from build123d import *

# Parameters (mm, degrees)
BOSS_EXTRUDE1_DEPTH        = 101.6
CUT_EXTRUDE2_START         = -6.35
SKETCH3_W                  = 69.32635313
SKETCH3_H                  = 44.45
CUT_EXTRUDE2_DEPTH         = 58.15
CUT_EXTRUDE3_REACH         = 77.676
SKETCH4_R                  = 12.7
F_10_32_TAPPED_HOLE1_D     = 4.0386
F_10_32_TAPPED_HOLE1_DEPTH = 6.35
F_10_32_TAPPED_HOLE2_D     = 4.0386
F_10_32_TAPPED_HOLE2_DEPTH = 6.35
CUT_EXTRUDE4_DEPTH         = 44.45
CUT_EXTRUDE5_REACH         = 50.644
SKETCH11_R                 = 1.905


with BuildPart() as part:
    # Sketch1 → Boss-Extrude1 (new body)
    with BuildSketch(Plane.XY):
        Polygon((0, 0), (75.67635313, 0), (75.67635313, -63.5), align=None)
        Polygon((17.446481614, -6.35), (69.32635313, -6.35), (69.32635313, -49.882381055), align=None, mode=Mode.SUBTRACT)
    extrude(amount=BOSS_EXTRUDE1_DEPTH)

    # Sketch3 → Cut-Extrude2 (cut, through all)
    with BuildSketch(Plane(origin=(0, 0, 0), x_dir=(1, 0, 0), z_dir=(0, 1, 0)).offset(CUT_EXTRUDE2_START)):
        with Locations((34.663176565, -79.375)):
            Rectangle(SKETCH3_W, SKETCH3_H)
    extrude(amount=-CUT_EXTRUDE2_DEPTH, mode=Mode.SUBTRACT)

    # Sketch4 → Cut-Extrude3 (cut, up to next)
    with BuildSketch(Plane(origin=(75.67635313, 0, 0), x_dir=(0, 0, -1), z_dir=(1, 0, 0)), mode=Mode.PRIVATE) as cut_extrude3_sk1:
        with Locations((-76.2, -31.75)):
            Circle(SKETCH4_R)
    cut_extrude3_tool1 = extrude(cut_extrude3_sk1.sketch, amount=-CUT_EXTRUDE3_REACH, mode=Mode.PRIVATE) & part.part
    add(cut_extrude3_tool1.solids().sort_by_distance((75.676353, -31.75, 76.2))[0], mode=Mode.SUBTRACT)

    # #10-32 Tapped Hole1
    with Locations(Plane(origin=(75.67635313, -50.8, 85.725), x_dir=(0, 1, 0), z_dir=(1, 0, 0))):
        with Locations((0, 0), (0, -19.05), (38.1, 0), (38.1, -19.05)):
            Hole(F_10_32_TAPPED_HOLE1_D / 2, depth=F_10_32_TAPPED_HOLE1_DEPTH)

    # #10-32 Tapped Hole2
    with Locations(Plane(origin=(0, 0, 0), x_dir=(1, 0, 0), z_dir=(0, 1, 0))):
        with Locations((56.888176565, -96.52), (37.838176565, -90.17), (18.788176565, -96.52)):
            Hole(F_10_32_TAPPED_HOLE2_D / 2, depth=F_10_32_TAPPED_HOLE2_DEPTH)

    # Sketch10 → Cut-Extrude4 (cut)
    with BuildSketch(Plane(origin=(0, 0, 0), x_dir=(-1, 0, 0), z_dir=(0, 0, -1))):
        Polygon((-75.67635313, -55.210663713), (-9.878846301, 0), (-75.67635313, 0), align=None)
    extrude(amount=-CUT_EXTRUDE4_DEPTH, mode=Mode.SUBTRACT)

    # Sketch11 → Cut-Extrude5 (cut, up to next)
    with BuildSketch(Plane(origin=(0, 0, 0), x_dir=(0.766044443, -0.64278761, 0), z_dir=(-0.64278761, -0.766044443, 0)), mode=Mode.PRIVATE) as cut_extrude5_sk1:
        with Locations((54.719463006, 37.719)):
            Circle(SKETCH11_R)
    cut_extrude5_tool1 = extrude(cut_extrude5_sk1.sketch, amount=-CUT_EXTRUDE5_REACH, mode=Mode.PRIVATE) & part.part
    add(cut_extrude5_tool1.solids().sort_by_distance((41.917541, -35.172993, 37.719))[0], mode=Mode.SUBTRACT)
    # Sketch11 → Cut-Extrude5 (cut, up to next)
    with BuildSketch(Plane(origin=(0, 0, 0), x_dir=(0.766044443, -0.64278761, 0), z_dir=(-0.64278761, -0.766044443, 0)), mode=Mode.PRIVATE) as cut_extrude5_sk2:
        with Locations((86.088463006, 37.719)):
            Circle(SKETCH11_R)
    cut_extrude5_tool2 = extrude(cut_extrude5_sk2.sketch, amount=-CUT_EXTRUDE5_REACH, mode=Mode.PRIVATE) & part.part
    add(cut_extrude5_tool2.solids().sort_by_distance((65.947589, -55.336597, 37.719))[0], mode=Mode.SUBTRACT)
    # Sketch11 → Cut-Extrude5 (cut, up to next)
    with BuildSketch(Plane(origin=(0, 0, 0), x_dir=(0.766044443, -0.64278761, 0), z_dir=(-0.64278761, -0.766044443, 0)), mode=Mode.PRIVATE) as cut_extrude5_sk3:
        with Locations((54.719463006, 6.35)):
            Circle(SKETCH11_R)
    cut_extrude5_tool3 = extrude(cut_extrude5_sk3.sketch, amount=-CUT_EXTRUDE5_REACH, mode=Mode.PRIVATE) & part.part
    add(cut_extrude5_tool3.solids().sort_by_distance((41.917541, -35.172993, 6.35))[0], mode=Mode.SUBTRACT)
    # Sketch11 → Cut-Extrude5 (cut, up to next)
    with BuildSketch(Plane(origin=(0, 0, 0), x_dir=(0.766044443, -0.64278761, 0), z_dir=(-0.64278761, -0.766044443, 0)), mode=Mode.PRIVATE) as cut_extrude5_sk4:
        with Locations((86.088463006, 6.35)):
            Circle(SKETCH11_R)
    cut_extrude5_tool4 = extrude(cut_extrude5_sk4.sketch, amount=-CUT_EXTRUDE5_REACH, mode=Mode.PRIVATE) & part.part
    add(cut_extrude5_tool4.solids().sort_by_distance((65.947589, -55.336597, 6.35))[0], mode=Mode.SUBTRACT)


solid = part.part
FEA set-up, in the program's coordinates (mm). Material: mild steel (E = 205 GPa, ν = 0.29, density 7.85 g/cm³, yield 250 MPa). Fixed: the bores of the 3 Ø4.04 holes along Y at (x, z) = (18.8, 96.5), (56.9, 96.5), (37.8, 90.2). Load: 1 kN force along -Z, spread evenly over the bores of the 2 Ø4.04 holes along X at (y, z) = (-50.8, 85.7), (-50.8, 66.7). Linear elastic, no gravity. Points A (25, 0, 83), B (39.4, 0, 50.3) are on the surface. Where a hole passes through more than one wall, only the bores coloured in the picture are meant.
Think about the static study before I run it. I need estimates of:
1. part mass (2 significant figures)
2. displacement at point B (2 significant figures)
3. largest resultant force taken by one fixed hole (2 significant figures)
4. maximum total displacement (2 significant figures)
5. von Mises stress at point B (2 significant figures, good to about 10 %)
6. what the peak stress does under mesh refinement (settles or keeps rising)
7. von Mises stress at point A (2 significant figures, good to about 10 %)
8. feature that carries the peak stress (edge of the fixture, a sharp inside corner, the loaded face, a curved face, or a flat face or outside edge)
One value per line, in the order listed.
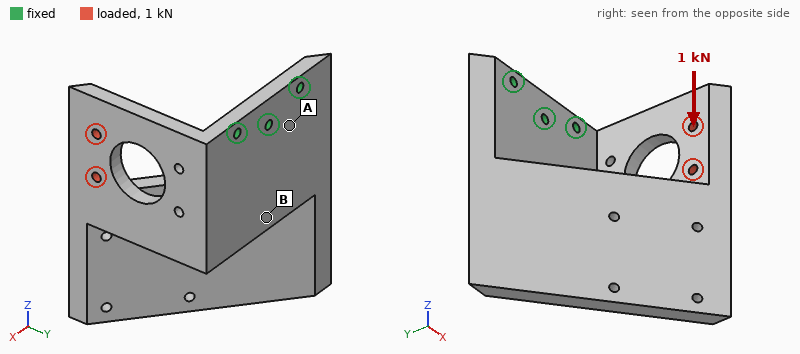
580 g
0.082 mm
1.3 kN
0.34 mm
20 MPa
keeps rising
56 MPa
edge of the fixture
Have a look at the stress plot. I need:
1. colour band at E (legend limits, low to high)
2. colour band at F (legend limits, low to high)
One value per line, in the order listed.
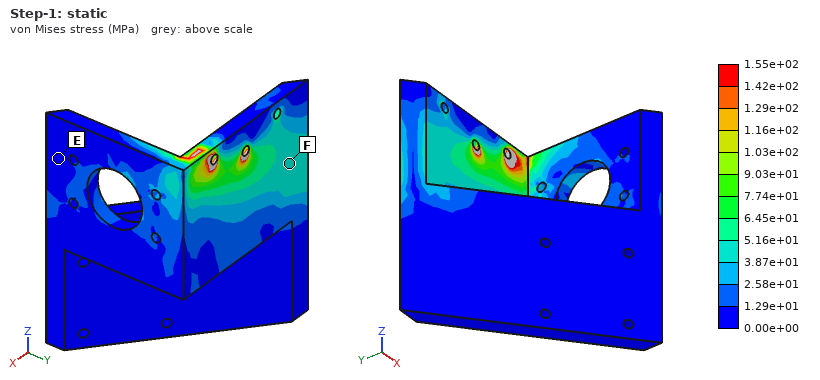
0.00e+00 to 1.29e+01 MPa
3.87e+01 to 5.16e+01 MPa
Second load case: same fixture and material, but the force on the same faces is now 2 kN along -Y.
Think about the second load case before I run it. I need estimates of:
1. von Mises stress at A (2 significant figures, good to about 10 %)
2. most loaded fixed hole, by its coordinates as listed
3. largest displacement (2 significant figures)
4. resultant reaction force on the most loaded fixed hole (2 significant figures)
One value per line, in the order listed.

44 MPa
(56.9, 96.5)
0.27 mm
2.0 kN
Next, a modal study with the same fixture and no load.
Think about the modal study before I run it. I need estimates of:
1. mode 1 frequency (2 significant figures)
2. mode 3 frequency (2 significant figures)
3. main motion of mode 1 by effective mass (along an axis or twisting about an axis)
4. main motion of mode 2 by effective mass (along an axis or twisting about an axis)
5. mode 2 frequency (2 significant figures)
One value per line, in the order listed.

520 Hz
1600 Hz
along Y
along X
1100 Hz
